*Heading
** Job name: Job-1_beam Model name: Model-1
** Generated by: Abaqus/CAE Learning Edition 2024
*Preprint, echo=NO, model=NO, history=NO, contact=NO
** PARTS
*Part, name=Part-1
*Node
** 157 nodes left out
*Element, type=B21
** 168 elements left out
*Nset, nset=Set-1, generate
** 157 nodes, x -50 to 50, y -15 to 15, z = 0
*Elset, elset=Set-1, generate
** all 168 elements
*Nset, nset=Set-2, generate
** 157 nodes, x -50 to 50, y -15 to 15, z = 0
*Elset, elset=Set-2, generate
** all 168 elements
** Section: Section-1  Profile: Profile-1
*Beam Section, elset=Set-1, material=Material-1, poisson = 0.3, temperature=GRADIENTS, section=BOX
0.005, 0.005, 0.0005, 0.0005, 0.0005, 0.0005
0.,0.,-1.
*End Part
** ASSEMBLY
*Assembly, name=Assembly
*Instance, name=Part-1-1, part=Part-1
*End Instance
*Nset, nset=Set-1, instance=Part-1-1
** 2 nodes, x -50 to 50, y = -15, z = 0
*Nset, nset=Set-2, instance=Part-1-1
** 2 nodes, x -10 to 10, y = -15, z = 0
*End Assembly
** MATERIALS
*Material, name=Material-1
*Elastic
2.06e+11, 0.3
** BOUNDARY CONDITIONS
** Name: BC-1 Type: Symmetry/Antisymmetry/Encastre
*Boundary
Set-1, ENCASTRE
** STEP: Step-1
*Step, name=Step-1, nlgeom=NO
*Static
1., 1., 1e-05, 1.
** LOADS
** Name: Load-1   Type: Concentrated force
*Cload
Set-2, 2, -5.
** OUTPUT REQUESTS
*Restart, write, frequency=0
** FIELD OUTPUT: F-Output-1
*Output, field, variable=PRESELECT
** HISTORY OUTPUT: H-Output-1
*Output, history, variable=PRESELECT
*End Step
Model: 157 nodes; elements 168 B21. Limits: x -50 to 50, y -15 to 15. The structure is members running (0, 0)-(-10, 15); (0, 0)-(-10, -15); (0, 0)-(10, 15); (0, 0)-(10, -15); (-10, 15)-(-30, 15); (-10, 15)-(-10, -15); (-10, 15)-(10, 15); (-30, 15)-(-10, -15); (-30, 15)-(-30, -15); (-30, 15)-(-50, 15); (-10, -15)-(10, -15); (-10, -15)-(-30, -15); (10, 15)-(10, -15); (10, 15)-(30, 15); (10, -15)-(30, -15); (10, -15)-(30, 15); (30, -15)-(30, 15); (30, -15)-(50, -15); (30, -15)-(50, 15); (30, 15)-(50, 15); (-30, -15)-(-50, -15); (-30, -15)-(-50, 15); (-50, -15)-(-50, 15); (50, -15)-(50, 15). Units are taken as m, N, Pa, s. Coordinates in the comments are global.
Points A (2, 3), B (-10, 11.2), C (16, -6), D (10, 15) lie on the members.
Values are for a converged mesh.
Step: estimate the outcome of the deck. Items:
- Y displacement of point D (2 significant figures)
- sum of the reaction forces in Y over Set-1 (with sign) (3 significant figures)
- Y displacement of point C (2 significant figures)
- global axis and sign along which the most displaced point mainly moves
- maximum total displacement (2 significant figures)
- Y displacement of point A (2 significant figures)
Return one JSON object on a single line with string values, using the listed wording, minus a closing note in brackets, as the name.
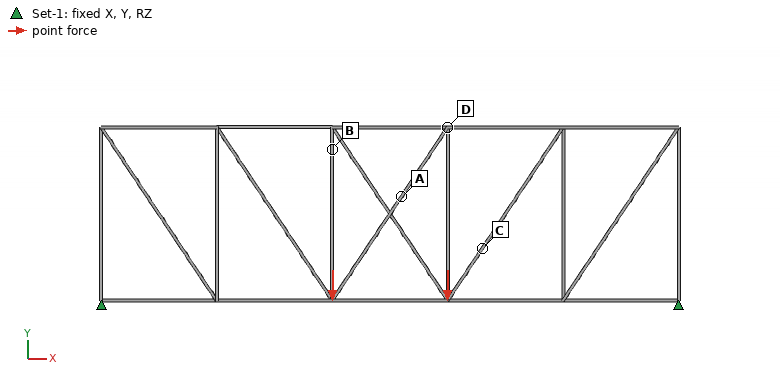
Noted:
{"Y displacement of point D": "-6.4e-04 m", "sum of the reaction forces in Y over Set-1 (with sign)": "10.0 N", "Y displacement of point C": "-5.9e-04 m", "global axis and sign along which the most displaced point mainly moves": "-Y", "maximum total displacement": "6.7e-04 m", "Y displacement of point A": "-6.6e-04 m"}
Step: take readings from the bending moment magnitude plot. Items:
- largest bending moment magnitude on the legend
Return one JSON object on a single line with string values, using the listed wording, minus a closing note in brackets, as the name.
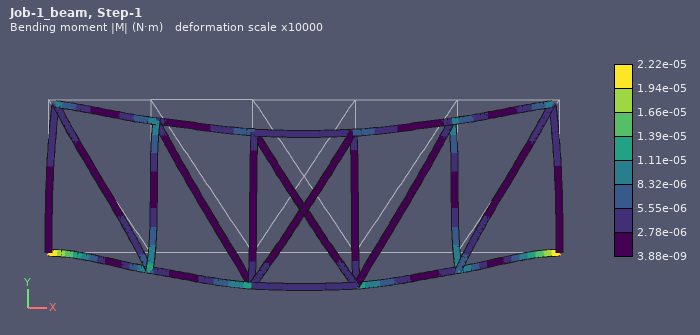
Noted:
{"largest bending moment magnitude on the legend": "2.22e-05 N·m"}
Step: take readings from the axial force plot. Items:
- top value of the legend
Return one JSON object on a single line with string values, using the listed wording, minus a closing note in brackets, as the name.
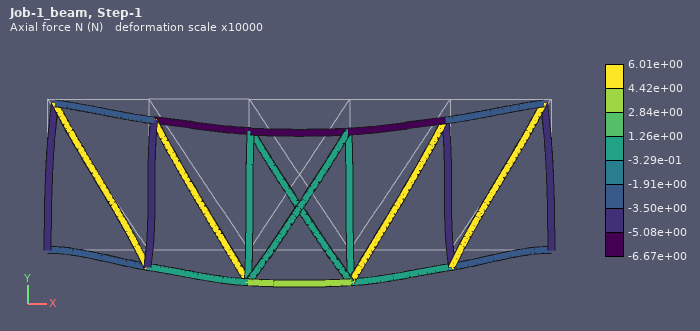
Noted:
{"top value of the legend": "6.01e+00 N"}
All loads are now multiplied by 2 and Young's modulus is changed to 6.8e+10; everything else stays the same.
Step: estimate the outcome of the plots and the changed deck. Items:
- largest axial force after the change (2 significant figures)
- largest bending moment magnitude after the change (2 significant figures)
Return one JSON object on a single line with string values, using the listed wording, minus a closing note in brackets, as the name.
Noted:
{"largest axial force after the change": "12 N", "largest bending moment magnitude after the change": "4.4e-05 N·m"}
